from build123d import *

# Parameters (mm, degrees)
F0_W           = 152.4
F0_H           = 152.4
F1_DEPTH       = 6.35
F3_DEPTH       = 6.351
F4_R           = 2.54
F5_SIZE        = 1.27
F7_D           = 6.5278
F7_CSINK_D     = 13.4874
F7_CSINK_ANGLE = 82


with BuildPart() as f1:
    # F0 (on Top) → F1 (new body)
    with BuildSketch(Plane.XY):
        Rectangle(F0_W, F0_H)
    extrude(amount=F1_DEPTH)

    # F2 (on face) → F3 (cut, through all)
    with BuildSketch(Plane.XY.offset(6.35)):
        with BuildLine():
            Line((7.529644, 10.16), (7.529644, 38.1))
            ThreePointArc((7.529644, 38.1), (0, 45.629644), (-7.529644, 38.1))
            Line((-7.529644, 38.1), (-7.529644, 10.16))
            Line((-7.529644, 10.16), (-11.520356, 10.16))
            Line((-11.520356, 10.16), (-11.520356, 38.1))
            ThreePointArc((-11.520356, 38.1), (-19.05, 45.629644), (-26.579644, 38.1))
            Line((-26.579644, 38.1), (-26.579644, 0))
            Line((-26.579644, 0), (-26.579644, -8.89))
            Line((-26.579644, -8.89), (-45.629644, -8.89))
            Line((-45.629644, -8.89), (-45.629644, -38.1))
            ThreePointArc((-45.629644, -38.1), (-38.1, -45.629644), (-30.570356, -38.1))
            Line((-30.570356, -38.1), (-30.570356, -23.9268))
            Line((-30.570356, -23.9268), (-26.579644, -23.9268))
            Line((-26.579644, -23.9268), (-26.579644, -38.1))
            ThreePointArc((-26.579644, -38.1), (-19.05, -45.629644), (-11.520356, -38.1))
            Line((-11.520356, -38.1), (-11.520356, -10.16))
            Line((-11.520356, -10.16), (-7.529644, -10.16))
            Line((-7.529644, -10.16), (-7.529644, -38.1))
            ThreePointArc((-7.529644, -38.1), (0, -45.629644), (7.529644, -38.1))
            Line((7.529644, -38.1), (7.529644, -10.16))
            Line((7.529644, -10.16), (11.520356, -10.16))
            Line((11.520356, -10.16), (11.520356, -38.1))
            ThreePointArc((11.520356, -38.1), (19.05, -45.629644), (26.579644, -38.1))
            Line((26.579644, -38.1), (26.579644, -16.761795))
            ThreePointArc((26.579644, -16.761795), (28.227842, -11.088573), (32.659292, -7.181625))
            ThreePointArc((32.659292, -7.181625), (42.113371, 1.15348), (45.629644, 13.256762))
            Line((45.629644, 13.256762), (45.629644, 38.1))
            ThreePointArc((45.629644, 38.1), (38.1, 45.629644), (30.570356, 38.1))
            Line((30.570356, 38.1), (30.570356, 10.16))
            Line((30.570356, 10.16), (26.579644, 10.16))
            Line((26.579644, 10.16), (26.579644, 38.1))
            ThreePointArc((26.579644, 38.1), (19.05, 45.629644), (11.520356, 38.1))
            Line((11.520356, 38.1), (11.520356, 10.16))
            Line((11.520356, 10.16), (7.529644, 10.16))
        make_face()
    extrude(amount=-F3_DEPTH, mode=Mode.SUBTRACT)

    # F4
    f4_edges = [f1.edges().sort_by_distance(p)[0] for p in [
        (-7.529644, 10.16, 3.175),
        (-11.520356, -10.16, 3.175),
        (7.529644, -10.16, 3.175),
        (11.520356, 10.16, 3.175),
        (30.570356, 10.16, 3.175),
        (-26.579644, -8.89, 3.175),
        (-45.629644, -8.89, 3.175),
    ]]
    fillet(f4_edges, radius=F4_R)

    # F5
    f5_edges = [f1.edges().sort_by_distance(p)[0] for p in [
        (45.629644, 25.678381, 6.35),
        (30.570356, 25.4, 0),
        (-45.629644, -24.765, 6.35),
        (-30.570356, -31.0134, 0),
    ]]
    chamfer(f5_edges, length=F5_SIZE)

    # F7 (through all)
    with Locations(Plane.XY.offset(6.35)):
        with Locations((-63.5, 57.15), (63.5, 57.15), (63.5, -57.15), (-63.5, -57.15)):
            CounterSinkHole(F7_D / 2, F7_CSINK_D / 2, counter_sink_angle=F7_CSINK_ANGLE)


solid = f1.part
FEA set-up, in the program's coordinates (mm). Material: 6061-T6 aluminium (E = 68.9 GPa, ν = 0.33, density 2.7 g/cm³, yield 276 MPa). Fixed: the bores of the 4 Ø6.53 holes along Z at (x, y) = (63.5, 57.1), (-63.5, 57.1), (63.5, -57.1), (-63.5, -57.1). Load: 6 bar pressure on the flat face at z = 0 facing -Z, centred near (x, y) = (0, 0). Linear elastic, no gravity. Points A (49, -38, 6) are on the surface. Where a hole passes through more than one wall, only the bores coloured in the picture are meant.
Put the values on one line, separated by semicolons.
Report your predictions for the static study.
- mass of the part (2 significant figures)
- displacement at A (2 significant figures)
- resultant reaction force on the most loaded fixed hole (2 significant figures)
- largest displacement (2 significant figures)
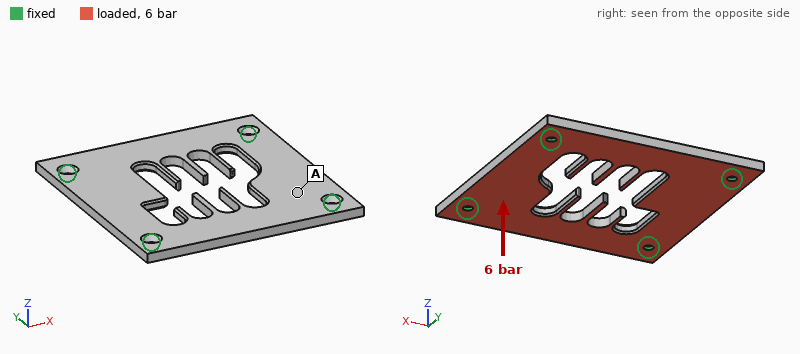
300 g; 0.26 mm; 4.0 kN; 0.99 mm
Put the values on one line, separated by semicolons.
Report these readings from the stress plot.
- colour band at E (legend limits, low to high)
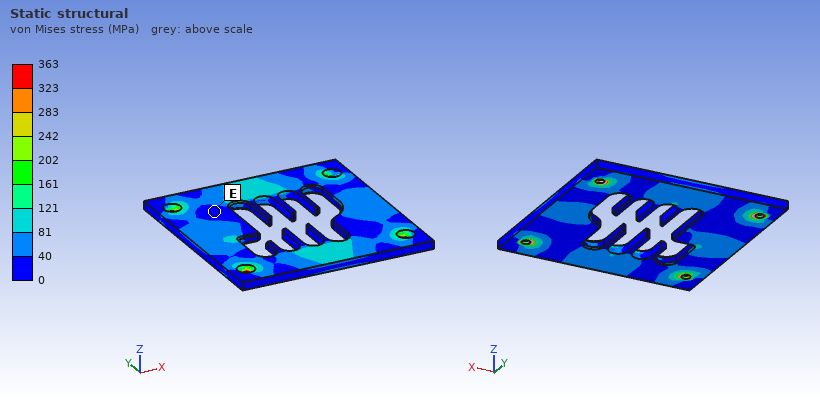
0 to 40 MPa
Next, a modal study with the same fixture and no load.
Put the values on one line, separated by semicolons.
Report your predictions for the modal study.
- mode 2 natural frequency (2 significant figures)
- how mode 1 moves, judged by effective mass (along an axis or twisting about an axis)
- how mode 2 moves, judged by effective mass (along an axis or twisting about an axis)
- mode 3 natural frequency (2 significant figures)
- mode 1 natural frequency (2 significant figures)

1600 Hz; along Z; twisting about X; 1900 Hz; 1400 Hz
